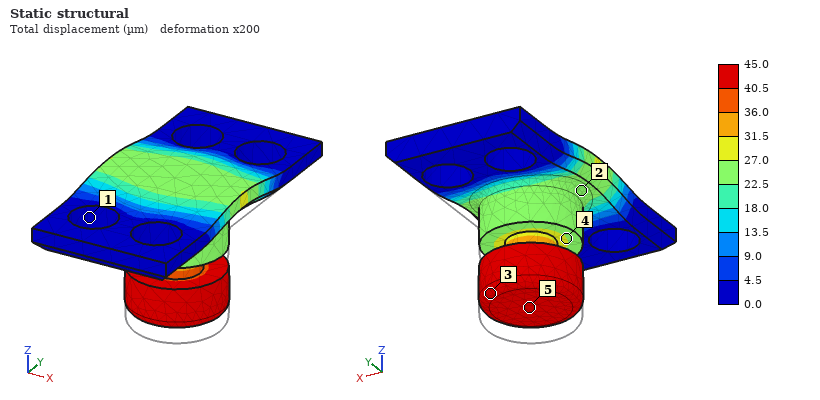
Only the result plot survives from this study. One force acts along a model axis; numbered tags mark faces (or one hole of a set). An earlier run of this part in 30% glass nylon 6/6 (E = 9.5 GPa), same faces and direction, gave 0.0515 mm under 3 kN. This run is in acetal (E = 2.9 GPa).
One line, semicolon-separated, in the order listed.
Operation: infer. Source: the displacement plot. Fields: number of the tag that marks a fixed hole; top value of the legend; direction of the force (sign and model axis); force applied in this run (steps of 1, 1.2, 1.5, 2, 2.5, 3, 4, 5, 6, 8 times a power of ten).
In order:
1; 45.0 µm; +Z; 800 N
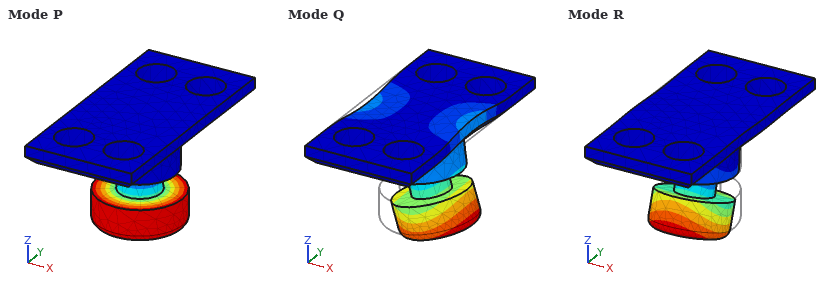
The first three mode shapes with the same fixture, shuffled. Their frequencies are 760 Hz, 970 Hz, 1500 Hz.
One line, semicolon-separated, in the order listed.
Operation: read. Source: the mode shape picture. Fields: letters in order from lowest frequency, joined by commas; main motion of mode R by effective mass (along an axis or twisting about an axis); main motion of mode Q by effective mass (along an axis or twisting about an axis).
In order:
Q, R, P; along Y; along X
